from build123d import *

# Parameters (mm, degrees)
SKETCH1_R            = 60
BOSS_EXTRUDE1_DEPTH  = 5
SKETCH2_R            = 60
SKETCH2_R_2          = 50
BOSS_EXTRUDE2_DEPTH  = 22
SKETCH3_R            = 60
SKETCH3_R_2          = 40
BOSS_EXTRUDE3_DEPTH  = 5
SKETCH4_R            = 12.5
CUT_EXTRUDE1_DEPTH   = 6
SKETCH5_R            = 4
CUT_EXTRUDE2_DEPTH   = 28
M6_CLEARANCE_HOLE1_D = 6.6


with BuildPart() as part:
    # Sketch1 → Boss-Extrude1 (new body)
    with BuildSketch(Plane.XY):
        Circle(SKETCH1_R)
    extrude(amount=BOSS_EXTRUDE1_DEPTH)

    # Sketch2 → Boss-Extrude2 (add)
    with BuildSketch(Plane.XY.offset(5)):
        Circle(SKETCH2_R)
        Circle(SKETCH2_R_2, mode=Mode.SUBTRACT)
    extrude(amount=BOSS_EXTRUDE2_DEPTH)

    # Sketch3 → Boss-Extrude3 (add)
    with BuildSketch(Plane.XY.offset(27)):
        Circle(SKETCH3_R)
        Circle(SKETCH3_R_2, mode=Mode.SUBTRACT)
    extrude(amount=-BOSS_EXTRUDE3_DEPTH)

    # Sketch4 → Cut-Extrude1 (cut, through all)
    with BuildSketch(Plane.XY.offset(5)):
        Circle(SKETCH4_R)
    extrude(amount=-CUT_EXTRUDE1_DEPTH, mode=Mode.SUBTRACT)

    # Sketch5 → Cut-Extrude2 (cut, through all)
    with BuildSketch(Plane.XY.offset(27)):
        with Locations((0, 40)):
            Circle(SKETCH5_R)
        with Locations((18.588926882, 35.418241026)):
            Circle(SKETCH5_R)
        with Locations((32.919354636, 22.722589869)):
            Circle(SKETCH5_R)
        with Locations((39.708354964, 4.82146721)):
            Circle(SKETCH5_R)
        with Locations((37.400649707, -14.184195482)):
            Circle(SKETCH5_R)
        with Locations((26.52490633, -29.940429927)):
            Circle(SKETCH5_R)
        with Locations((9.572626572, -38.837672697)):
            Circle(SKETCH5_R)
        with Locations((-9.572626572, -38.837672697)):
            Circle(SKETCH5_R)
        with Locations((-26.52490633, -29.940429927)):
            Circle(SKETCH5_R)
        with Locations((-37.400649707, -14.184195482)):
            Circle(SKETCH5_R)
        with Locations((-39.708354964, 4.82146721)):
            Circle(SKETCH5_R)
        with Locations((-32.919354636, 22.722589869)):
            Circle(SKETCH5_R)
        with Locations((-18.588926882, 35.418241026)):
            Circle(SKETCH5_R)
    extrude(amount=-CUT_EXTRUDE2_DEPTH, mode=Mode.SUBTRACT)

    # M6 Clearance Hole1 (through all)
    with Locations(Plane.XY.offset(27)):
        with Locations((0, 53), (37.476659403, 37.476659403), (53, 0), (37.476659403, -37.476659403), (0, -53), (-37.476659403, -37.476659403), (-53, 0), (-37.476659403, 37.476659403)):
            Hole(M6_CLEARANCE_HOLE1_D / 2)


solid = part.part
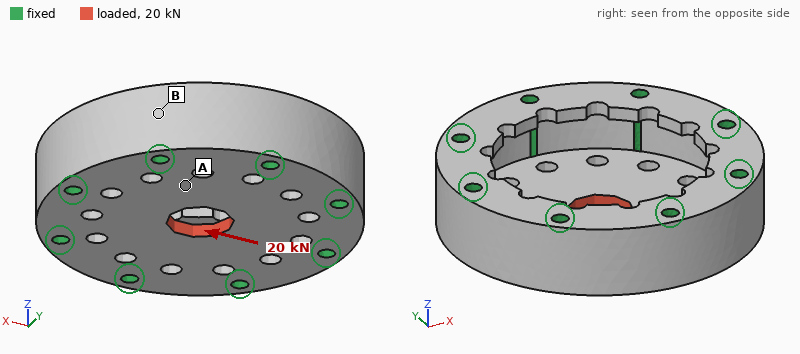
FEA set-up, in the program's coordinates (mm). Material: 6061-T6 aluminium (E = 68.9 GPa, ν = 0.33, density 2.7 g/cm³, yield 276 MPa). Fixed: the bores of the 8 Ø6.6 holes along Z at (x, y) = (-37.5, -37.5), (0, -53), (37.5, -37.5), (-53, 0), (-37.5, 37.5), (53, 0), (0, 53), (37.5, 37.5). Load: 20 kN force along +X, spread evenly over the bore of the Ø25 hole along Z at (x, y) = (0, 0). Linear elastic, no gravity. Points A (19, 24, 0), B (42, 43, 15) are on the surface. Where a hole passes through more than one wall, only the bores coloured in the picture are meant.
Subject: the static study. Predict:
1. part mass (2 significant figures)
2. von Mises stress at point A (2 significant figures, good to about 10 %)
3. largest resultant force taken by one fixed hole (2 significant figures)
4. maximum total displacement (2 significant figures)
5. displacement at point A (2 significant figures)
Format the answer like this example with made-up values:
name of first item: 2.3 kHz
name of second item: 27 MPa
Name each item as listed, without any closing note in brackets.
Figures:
part mass: 360 g
von Mises stress at point A: 31 MPa
largest resultant force taken by one fixed hole: 4.0 kN
maximum total displacement: 27 µm
displacement at point A: 11 µm
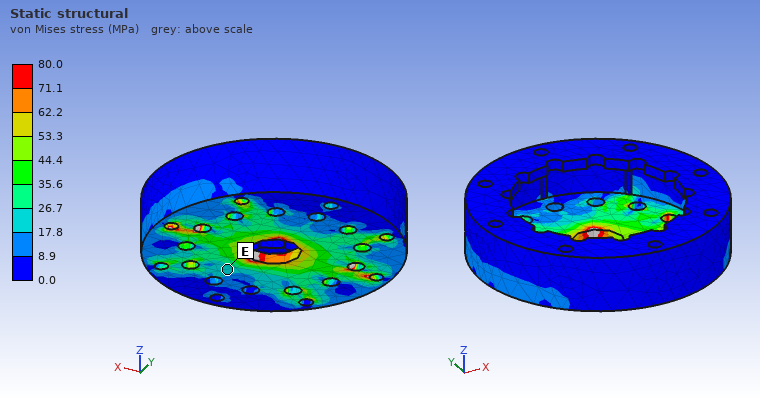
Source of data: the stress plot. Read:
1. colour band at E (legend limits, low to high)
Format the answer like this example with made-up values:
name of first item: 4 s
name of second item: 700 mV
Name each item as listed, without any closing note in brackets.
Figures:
colour band at E: 17.8 to 26.7 MPa
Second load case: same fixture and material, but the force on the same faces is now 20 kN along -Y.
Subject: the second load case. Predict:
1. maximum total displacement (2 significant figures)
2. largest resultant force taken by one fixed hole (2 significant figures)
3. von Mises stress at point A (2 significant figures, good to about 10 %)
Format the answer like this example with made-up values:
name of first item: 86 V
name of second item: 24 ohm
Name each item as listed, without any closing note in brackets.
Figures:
maximum total displacement: 27 µm
largest resultant force taken by one fixed hole: 4.1 kN
von Mises stress at point A: 32 MPa
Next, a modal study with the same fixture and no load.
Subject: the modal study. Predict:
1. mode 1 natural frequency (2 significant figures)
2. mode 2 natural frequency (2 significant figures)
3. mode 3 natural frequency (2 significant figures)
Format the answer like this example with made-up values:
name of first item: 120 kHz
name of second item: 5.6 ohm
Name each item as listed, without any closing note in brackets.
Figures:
mode 1 natural frequency: 4500 Hz
mode 2 natural frequency: 8400 Hz
mode 3 natural frequency: 8400 Hz
